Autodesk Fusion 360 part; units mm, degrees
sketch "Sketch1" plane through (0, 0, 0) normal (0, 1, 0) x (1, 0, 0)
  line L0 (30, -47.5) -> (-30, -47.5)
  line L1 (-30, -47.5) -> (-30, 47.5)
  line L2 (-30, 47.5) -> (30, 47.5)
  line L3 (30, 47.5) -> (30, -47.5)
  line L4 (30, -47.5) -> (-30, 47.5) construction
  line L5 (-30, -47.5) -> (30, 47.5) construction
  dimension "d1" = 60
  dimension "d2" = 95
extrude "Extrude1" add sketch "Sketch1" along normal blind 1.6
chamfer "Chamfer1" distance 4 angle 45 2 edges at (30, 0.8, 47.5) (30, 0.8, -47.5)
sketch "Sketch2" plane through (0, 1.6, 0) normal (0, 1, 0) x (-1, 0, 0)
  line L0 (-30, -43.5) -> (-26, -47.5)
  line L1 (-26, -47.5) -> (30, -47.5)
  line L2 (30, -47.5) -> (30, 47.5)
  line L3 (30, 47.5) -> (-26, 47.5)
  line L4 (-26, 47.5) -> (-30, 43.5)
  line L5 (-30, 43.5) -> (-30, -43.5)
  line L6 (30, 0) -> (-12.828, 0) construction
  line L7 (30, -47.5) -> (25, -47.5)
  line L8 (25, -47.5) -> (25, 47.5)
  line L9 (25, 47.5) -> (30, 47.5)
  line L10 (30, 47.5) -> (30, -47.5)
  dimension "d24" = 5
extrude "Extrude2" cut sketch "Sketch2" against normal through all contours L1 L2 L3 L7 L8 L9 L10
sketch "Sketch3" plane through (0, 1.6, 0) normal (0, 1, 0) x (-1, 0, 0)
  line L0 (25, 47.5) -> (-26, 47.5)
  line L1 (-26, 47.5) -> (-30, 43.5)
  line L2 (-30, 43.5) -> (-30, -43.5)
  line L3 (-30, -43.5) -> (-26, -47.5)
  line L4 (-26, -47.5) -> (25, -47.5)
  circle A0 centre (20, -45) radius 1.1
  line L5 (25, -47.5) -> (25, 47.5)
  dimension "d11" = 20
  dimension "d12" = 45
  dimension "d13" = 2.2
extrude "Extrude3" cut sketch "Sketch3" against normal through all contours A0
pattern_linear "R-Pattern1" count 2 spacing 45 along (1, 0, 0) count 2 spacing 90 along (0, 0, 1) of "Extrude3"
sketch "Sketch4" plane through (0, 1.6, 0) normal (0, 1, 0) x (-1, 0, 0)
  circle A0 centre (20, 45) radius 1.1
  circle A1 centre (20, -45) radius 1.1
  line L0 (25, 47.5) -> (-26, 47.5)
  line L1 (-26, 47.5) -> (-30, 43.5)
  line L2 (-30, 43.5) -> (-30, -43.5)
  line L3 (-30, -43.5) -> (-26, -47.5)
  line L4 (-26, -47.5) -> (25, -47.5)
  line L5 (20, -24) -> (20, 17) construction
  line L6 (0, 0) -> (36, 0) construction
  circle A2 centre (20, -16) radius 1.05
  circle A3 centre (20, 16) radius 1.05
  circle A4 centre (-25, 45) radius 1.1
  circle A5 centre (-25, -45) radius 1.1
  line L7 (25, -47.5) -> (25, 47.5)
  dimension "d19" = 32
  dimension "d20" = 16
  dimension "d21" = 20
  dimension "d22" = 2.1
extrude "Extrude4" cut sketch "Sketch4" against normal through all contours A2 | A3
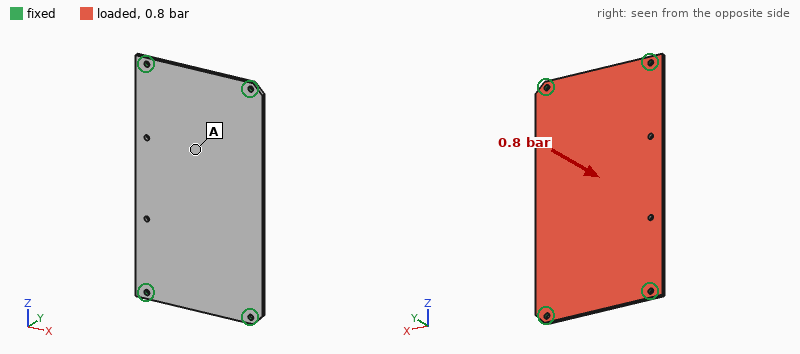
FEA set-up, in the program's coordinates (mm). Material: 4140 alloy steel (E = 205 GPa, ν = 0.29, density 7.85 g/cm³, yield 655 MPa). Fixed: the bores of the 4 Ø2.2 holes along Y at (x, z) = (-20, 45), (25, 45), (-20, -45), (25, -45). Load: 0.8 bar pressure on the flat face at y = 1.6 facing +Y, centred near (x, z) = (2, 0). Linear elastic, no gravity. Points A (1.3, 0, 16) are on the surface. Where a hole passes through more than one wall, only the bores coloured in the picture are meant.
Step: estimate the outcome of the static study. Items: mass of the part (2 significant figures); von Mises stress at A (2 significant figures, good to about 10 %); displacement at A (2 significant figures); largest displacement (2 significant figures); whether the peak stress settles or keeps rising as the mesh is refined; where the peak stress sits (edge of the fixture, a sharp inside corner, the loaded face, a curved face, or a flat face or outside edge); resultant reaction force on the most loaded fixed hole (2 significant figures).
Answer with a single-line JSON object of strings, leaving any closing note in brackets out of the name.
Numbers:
{"mass of the part": "65 g", "von Mises stress at A": "47 MPa", "displacement at A": "0.23 mm", "largest displacement": "0.28 mm", "whether the peak stress settles or keeps rising as the mesh is refined": "keeps rising", "where the peak stress sits": "edge of the fixture", "resultant reaction force on the most loaded fixed hole": "100 N"}
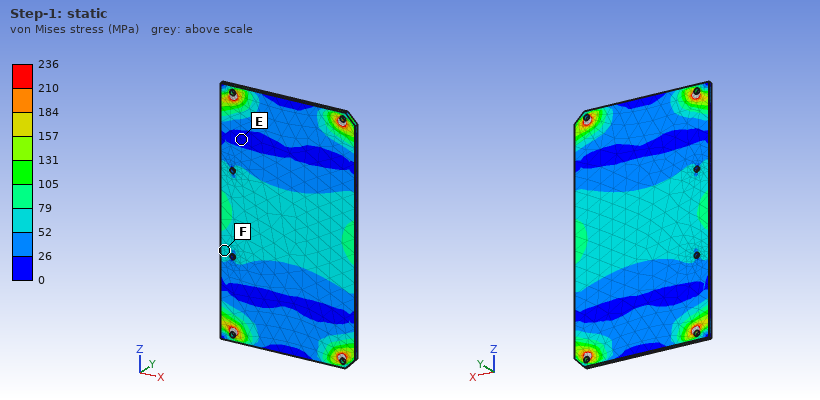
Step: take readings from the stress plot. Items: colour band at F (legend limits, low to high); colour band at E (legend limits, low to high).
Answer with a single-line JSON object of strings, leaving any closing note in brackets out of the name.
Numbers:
{"colour band at F": "52 to 79 MPa", "colour band at E": "0 to 26 MPa"}
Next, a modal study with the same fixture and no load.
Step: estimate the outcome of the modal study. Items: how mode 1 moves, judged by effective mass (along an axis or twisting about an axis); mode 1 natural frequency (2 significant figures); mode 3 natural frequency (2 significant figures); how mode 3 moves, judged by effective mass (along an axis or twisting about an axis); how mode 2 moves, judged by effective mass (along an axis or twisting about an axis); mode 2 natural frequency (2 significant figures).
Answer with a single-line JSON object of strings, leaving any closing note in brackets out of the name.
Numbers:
{"how mode 1 moves, judged by effective mass": "along Y", "mode 1 natural frequency": "860 Hz", "mode 3 natural frequency": "2400 Hz", "how mode 3 moves, judged by effective mass": "twisting about X", "how mode 2 moves, judged by effective mass": "twisting about Z", "mode 2 natural frequency": "1500 Hz"}
